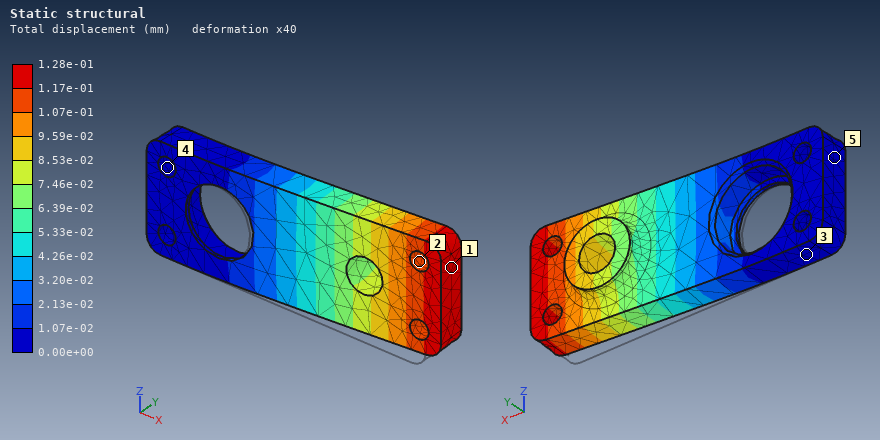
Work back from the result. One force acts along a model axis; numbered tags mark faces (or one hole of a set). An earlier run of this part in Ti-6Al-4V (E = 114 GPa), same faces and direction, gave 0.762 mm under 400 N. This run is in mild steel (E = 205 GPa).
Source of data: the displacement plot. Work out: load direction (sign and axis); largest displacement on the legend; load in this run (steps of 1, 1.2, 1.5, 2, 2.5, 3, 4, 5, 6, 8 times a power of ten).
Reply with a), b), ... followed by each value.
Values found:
a) +Y
b) 1.28e-01 mm
c) 120 N
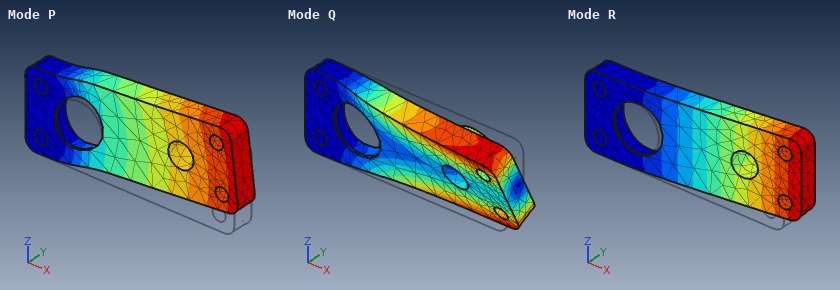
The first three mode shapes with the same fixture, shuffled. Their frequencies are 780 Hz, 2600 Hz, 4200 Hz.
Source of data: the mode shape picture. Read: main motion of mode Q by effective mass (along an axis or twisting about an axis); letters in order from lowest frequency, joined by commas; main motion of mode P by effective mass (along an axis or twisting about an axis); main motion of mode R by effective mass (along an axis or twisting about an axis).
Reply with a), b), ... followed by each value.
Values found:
a) twisting about X
b) R, P, Q
c) along Z
d) along Y
